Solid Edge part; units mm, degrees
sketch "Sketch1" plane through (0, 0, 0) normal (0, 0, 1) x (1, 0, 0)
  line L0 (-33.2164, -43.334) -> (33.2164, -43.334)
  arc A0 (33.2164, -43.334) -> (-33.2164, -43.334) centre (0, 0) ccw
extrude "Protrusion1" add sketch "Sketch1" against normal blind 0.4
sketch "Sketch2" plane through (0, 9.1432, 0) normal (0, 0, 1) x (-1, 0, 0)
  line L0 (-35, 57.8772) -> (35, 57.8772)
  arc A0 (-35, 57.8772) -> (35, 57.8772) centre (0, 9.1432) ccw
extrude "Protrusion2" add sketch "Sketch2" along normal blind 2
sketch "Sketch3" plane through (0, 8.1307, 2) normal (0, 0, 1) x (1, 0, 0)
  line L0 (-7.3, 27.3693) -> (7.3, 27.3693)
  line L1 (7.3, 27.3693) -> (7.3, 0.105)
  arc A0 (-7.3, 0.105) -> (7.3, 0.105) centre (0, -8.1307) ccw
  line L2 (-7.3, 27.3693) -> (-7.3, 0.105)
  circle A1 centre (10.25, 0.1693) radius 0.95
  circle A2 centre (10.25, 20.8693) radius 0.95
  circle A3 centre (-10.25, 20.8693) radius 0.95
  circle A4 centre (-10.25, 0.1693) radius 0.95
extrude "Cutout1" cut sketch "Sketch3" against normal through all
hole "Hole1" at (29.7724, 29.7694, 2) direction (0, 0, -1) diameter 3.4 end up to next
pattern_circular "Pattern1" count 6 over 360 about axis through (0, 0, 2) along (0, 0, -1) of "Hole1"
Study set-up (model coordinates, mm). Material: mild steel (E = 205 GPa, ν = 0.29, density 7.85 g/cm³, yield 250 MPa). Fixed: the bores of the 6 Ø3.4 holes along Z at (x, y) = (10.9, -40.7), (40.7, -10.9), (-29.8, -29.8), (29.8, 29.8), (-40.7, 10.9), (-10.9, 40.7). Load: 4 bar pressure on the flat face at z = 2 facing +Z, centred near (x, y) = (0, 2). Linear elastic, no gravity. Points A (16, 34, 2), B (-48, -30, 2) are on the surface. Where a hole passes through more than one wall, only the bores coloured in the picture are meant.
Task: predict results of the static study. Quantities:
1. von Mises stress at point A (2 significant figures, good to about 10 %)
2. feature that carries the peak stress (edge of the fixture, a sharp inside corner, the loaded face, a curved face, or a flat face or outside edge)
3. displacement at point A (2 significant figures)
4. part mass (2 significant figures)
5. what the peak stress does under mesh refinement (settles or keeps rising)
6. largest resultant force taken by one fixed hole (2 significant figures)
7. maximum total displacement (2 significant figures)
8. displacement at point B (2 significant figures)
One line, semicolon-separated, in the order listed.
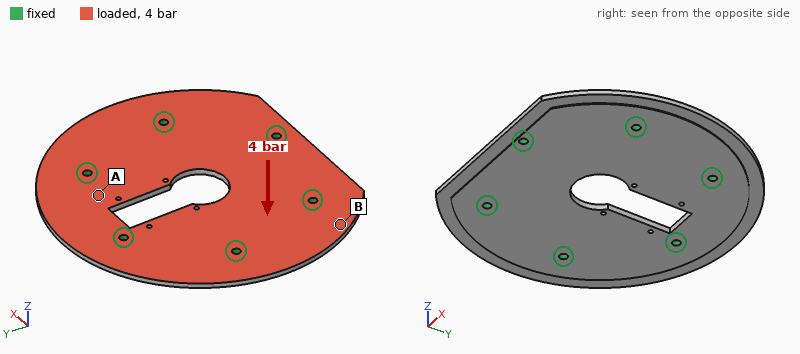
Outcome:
64 MPa; edge of the fixture; 18 µm; 180 g; keeps rising; 730 N; 74 µm; 31 µm
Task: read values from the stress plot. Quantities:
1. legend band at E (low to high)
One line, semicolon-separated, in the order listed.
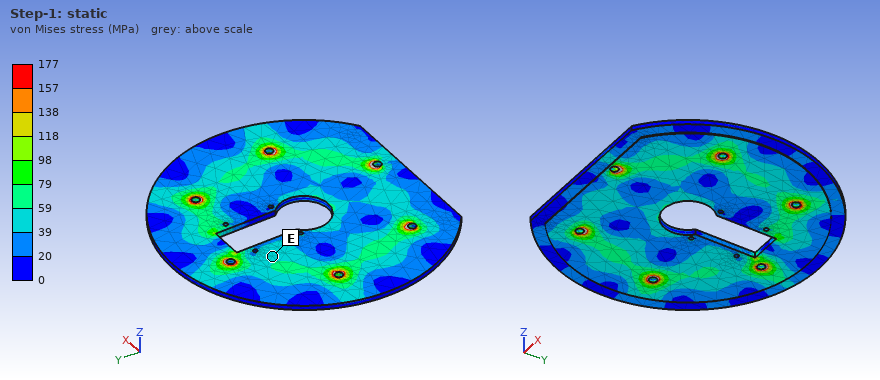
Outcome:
39 to 59 MPa
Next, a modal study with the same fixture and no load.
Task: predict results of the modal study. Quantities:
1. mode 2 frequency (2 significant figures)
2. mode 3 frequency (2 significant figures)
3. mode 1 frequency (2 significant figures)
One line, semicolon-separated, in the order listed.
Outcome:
3400 Hz; 3500 Hz; 2900 Hz
